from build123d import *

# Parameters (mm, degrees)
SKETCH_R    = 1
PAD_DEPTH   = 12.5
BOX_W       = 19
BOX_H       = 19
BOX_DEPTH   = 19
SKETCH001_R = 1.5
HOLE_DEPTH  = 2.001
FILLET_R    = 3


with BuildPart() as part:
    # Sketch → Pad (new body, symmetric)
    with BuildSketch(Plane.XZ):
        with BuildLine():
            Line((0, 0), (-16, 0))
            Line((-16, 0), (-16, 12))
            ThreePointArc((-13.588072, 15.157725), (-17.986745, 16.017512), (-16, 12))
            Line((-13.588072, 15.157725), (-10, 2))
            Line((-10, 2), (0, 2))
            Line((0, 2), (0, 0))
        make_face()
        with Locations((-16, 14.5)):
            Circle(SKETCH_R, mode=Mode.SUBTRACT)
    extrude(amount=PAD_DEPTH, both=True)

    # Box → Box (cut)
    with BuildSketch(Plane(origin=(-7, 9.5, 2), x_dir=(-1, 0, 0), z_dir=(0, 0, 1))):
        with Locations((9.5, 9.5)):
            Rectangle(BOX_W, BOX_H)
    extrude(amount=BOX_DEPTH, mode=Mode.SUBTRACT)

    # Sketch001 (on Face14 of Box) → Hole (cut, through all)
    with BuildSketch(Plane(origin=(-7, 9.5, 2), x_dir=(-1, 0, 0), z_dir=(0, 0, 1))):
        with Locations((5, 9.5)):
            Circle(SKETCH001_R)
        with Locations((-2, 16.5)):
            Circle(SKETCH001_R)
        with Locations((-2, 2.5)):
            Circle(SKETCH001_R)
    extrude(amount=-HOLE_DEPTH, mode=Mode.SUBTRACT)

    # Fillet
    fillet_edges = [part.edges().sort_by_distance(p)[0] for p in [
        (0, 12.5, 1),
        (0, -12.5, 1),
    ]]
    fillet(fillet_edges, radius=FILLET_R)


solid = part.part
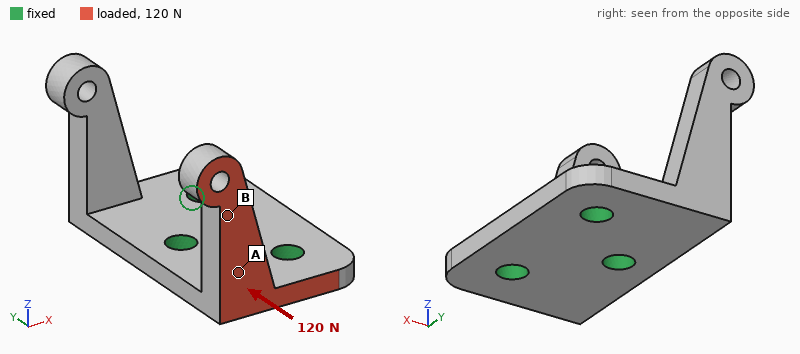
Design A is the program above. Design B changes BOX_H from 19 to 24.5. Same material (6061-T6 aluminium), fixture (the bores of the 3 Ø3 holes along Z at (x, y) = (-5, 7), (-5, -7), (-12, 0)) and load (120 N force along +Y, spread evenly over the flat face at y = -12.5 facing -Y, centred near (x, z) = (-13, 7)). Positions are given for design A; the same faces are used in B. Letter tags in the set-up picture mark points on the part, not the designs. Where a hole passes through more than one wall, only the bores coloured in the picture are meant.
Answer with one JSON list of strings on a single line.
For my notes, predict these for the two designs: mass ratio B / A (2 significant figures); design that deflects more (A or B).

["0.69", "B"]
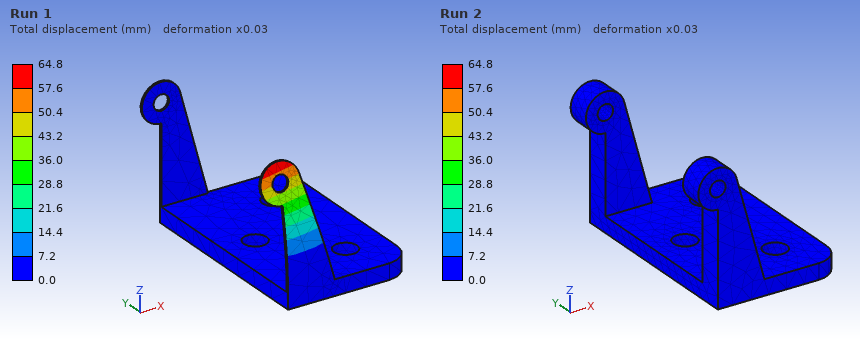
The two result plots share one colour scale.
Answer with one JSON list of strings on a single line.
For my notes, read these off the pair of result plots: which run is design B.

["Run 1"]
